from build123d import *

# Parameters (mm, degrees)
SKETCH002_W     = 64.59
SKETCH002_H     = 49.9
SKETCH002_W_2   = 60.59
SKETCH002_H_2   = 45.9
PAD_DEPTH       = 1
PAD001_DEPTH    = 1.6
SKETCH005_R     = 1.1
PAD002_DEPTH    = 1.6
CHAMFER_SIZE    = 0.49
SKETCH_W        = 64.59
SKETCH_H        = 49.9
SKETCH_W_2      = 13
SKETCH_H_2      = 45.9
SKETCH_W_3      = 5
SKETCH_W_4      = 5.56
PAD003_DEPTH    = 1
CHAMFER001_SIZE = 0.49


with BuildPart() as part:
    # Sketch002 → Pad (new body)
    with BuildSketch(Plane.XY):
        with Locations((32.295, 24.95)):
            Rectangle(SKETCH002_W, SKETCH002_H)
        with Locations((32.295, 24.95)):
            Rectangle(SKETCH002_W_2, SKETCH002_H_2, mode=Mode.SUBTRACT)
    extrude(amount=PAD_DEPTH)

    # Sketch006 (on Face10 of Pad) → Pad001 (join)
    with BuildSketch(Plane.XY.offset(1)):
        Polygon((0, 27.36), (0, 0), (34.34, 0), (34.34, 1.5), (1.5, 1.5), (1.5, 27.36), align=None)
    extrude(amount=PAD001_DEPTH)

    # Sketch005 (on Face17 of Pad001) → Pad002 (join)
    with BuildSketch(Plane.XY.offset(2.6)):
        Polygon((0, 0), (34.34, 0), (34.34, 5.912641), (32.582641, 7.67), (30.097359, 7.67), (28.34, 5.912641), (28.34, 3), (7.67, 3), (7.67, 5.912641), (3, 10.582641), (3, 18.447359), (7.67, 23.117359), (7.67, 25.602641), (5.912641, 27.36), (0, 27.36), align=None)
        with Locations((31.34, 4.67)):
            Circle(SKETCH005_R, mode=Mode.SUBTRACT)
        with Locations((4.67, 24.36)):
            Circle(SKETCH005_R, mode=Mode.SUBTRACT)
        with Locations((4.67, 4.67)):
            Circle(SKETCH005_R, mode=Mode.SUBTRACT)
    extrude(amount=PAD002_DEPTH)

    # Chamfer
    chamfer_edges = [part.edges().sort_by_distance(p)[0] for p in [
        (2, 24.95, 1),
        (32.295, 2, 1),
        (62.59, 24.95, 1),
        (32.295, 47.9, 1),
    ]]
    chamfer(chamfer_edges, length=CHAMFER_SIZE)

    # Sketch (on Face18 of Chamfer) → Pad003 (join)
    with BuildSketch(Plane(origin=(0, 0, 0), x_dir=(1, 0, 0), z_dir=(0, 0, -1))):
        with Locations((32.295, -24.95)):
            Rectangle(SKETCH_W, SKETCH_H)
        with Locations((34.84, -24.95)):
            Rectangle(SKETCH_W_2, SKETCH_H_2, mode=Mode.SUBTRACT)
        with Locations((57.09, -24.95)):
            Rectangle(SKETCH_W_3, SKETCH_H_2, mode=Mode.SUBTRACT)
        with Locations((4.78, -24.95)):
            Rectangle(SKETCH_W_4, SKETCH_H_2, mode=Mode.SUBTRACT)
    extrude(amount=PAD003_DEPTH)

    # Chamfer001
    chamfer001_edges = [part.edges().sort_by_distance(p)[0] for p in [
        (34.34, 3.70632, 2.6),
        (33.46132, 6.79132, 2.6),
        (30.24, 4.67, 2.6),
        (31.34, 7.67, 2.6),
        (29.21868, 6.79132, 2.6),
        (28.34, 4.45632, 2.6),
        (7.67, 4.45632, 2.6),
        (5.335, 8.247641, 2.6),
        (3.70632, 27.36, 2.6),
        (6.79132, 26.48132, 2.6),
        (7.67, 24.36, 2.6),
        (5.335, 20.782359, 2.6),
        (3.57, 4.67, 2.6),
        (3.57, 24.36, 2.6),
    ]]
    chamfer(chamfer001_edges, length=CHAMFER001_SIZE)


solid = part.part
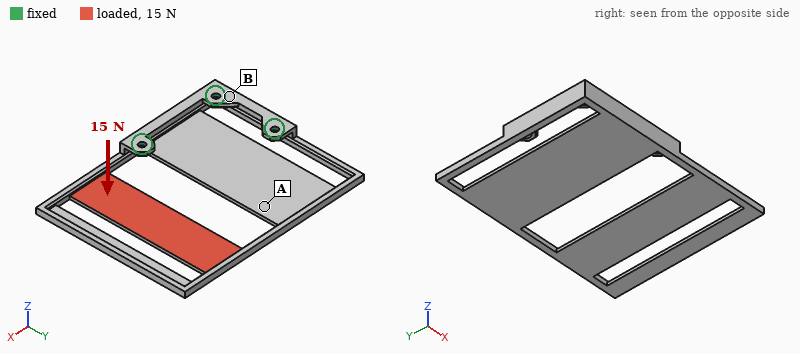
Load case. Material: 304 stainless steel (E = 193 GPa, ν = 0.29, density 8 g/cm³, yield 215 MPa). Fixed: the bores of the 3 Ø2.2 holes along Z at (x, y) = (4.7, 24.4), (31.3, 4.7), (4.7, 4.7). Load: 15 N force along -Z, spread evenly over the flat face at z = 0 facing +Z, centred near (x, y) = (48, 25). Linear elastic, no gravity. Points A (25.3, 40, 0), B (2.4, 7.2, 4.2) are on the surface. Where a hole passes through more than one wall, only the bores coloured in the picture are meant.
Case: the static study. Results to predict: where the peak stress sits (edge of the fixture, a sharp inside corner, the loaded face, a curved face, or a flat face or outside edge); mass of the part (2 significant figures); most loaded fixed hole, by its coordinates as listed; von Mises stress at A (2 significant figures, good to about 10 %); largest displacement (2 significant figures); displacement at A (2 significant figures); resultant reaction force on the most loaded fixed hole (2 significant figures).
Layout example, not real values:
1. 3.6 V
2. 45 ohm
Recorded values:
1. a flat face or outside edge
2. 25 g
3. (31.3, 4.7)
4. 34 MPa
5. 0.71 mm
6. 0.21 mm
7. 26 N
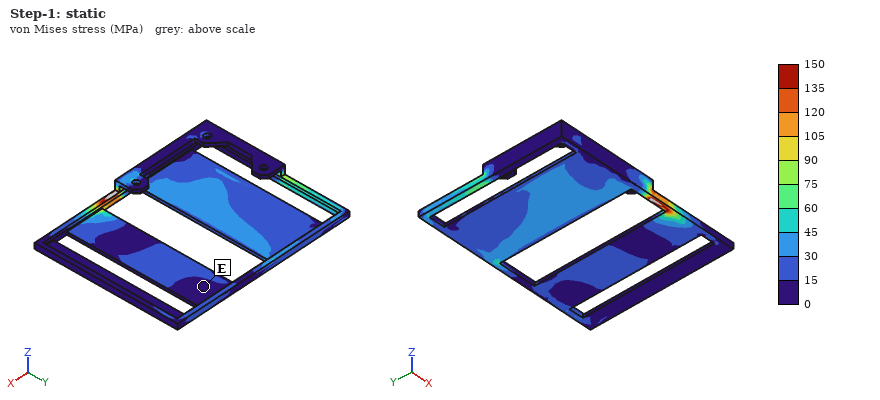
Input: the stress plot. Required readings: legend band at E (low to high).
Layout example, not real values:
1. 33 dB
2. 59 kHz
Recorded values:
1. 0 to 15 MPa
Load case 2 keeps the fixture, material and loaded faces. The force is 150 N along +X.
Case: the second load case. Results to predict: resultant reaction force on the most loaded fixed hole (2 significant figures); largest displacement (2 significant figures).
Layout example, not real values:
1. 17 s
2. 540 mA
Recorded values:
1. 130 N
2. 0.14 mm
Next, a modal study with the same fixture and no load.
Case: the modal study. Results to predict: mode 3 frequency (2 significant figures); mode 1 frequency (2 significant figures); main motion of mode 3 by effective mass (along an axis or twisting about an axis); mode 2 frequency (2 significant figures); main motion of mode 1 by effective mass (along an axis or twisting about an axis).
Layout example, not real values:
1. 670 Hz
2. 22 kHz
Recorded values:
1. 1300 Hz
2. 270 Hz
3. along Z
4. 740 Hz
5. along Z
